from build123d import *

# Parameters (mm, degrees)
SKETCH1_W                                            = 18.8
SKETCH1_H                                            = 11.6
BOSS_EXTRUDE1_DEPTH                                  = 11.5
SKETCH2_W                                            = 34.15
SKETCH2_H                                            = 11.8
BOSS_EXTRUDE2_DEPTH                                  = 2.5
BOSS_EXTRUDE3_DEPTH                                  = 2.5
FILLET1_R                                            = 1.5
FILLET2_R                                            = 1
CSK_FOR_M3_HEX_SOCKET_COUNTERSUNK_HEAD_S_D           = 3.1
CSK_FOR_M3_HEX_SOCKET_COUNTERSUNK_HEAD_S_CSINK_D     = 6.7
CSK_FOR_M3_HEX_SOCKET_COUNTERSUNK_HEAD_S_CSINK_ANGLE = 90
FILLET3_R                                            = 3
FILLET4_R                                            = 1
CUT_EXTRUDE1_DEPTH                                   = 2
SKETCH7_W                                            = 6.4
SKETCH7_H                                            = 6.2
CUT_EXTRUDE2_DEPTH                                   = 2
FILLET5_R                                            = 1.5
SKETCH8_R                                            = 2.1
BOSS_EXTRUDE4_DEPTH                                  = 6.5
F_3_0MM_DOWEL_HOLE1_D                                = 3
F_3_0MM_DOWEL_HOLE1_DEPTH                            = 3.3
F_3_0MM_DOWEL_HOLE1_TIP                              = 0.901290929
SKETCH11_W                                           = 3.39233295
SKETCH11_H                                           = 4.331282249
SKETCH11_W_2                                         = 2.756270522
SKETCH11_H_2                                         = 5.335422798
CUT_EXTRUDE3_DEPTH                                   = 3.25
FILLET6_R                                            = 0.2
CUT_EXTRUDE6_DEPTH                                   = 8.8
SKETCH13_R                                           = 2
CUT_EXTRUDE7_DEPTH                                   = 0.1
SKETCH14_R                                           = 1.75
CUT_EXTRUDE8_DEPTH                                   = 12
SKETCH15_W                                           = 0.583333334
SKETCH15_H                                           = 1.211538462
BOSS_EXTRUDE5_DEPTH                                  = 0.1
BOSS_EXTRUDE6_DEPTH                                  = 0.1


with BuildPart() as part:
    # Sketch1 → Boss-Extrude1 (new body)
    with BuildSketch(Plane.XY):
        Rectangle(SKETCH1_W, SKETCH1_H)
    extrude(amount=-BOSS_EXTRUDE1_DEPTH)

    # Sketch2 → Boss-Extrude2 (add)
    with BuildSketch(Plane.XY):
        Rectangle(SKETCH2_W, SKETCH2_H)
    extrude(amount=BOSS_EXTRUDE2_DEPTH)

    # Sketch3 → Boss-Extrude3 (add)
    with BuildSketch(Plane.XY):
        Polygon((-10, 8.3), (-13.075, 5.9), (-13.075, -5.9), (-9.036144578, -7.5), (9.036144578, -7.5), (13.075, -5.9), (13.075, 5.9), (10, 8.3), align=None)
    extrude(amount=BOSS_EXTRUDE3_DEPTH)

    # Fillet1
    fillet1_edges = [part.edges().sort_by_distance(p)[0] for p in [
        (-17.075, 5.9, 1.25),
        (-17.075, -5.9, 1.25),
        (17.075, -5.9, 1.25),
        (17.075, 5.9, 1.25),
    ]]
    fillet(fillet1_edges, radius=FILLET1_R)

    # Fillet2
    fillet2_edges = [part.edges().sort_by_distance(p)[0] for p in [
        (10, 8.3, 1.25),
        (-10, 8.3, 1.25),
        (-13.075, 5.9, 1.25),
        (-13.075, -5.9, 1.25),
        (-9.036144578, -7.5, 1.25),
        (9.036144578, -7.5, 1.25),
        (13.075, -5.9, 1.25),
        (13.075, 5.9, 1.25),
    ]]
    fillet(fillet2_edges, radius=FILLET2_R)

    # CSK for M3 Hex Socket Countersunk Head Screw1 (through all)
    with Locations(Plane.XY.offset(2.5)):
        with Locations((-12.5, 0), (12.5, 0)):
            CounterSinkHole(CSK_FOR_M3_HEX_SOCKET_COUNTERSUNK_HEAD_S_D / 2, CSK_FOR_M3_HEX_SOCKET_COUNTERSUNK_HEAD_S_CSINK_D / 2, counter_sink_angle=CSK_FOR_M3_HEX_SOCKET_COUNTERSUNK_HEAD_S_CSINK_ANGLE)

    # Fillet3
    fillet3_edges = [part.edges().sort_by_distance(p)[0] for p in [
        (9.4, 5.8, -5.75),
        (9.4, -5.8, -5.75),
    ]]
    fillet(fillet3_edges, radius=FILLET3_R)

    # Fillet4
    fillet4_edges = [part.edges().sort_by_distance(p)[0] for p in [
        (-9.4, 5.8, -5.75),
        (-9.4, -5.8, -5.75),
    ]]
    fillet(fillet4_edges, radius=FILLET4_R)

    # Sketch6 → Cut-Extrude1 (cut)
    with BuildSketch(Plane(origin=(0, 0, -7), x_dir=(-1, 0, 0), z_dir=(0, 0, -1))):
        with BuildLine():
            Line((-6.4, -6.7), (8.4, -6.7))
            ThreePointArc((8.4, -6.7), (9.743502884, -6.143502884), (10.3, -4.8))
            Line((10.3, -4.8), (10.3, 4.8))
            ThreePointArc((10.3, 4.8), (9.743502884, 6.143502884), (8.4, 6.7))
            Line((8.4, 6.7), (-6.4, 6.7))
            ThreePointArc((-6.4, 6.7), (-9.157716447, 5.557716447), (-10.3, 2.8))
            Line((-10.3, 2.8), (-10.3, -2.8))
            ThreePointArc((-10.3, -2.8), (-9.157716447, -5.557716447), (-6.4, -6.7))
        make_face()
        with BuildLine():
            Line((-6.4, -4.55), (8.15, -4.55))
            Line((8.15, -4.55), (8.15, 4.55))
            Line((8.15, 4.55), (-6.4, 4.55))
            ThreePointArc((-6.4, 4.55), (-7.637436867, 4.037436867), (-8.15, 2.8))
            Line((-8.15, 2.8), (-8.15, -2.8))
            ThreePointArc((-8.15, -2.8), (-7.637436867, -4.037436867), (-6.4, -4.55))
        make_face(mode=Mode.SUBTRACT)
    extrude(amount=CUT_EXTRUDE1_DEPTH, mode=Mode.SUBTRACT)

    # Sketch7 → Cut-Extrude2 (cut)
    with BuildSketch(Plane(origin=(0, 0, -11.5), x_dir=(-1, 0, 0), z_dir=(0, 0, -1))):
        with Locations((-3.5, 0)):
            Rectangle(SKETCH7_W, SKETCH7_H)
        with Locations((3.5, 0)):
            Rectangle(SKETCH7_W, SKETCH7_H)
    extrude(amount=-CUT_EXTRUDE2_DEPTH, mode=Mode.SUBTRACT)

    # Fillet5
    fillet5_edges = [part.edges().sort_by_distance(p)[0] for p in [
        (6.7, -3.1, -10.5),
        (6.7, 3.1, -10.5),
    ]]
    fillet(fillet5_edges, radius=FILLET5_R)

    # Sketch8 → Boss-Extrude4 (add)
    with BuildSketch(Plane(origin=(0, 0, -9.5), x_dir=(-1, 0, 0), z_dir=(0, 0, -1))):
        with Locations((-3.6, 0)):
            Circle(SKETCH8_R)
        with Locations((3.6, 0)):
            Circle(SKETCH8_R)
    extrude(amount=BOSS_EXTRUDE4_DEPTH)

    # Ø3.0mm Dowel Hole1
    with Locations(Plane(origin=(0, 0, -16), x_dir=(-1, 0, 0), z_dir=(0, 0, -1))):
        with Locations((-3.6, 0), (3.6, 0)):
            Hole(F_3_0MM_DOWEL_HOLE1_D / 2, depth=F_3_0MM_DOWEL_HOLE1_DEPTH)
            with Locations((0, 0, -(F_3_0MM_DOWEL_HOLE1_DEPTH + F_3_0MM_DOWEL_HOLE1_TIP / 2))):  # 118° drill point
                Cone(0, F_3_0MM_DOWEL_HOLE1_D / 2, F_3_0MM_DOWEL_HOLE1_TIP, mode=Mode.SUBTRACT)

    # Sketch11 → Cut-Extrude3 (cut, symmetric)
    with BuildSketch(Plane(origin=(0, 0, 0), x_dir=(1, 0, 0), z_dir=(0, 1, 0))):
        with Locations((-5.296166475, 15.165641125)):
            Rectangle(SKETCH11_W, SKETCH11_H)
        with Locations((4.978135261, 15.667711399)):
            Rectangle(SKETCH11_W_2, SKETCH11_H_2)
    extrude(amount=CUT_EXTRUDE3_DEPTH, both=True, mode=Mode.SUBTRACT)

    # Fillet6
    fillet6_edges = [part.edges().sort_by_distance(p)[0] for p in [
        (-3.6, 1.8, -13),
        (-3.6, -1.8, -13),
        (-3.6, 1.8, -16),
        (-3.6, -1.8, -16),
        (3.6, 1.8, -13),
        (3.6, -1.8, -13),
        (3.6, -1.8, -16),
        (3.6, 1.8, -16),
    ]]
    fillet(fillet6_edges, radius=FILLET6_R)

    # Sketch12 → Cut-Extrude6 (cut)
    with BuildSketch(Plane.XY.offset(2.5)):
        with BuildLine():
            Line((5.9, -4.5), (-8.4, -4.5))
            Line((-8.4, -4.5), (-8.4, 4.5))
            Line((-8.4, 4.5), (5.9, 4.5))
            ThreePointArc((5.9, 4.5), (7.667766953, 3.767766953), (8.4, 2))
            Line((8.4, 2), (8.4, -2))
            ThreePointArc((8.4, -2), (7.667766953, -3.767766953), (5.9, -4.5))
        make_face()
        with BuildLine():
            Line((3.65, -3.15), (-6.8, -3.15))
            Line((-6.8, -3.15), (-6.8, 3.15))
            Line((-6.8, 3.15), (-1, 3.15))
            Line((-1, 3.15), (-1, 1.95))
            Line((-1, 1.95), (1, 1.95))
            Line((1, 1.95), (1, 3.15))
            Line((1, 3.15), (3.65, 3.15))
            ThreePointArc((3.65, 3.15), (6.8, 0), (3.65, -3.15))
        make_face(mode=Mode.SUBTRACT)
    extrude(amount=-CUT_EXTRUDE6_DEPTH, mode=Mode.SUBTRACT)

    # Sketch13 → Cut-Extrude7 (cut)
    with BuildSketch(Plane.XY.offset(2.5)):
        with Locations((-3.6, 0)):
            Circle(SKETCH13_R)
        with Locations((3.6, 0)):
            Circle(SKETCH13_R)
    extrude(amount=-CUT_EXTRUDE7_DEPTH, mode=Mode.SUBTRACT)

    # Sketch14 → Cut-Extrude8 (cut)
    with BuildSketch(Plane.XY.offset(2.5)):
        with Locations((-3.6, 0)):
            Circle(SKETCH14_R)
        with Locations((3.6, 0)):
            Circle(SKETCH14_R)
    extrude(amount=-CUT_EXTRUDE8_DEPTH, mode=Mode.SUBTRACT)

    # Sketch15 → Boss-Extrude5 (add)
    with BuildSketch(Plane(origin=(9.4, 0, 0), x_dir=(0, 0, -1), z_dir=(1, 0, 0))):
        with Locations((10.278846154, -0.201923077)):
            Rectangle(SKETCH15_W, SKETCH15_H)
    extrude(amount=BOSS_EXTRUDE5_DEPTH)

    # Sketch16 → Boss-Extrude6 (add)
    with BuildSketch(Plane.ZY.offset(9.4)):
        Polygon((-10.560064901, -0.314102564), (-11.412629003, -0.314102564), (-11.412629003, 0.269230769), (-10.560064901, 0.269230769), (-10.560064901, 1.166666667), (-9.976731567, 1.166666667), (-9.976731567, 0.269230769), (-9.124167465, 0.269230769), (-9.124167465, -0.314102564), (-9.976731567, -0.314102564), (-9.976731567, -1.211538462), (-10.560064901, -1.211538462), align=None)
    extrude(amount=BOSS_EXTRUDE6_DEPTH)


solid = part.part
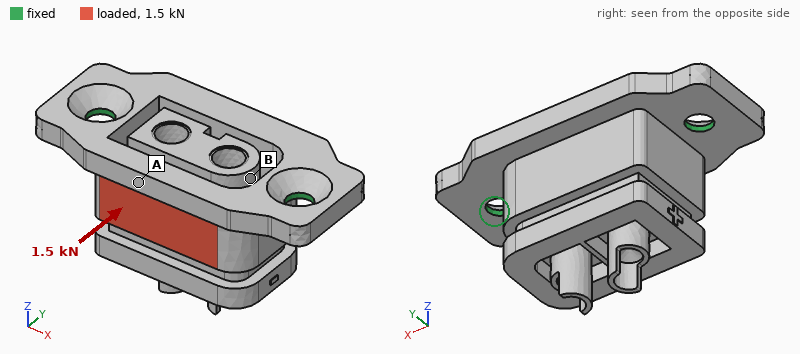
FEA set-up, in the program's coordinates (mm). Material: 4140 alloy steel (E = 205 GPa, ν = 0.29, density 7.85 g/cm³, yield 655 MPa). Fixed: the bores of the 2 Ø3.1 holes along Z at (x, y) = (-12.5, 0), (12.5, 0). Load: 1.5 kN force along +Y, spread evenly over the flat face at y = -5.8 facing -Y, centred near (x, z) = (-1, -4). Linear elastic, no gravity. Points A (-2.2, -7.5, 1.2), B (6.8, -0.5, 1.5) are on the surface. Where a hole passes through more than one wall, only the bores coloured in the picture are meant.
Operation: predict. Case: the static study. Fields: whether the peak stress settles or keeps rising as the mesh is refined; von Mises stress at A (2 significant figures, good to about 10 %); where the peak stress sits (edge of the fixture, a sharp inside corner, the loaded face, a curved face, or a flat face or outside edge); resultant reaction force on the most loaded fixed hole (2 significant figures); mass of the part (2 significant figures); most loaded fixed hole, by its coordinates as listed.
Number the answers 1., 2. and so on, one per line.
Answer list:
1. keeps rising
2. 160 MPa
3. edge of the fixture
4. 830 N
5. 20 g
6. (-12.5, 0)
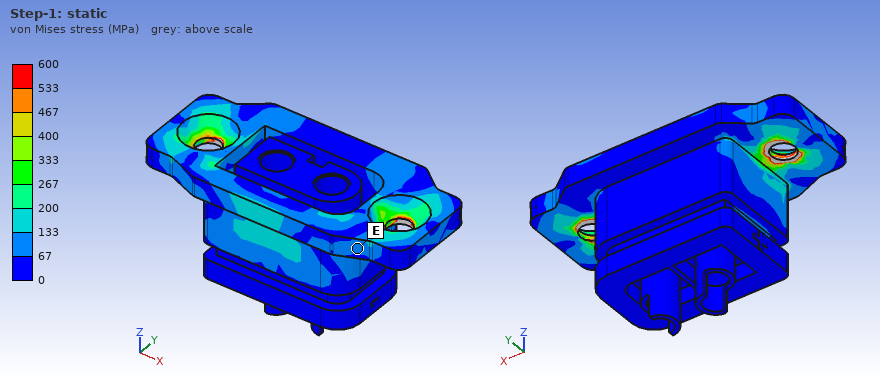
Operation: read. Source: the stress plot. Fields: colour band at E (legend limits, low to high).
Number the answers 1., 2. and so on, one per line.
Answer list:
1. 67 to 133 MPa
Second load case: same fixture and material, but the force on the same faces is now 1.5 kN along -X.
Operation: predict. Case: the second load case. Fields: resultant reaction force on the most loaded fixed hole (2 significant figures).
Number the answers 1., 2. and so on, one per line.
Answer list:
1. 850 N
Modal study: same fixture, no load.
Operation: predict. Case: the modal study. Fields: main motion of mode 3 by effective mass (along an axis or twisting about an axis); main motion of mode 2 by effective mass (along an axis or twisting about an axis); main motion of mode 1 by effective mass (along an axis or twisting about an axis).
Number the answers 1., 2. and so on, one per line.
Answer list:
1. along X
2. along Z
3. along Y
